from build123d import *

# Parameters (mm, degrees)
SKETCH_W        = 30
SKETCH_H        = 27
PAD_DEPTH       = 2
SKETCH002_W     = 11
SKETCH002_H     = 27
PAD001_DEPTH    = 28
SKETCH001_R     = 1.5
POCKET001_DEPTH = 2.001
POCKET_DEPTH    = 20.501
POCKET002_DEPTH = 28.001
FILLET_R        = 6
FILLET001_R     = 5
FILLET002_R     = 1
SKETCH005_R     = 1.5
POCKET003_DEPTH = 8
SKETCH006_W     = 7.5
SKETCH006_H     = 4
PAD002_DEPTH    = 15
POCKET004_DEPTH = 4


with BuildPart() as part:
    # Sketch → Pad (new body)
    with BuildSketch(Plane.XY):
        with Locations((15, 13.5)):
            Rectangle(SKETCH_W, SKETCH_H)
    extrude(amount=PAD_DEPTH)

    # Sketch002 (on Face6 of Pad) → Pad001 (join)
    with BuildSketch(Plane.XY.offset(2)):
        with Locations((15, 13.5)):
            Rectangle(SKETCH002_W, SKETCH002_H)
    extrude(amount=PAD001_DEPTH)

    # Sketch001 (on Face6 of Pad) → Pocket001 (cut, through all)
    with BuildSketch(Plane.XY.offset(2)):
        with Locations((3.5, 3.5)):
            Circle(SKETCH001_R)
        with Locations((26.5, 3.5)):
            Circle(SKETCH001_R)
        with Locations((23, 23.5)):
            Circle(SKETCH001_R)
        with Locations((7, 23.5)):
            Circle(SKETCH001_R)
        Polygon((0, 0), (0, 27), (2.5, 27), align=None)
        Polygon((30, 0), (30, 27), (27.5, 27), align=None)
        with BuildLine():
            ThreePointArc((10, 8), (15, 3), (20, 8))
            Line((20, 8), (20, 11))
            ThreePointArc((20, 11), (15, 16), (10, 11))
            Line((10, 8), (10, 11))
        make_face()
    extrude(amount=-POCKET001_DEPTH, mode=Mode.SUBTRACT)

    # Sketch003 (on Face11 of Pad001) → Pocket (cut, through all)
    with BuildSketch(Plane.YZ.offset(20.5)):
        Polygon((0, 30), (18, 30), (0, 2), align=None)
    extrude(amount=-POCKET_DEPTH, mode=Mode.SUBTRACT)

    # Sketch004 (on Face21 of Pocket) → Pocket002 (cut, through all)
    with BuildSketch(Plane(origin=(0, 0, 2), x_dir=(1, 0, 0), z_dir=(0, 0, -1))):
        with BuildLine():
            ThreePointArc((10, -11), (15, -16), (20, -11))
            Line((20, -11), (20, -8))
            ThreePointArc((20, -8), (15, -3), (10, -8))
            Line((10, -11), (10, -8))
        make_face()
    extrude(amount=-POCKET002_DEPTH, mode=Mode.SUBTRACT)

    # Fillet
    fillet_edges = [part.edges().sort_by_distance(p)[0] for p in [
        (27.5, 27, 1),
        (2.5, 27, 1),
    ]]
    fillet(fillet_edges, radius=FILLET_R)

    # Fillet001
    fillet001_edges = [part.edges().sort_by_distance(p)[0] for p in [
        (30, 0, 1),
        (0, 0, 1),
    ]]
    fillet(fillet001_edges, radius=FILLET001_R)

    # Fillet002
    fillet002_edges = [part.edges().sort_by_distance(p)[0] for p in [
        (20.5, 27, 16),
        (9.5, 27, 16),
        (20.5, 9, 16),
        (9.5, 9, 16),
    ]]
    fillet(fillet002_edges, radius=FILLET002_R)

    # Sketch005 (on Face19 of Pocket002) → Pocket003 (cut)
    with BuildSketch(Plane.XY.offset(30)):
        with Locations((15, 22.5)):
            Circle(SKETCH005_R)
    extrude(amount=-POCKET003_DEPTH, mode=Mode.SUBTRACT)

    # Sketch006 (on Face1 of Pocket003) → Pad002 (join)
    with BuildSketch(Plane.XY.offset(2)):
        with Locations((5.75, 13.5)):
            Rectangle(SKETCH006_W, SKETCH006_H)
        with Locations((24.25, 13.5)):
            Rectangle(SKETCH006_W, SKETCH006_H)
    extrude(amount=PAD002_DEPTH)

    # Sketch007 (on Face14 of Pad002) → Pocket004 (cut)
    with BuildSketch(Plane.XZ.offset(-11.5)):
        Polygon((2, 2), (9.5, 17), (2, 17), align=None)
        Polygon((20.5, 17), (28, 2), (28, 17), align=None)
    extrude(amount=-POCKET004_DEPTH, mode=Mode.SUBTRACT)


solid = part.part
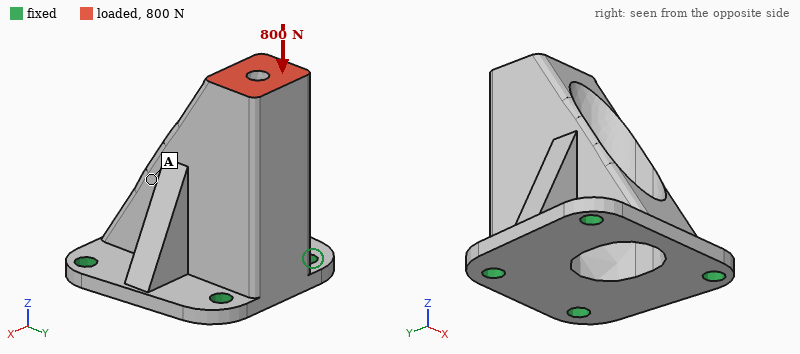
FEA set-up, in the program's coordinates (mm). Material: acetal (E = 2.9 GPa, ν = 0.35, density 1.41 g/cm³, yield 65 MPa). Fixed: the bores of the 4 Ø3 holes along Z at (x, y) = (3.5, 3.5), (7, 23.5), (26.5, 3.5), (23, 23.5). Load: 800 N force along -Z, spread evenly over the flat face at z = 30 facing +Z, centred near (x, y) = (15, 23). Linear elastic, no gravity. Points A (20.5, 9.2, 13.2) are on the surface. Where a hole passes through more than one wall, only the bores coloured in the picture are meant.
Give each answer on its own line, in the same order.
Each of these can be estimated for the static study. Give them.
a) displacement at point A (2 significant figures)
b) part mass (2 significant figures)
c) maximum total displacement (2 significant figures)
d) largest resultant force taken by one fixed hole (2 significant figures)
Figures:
0.073 mm
7.7 g
0.31 mm
410 N
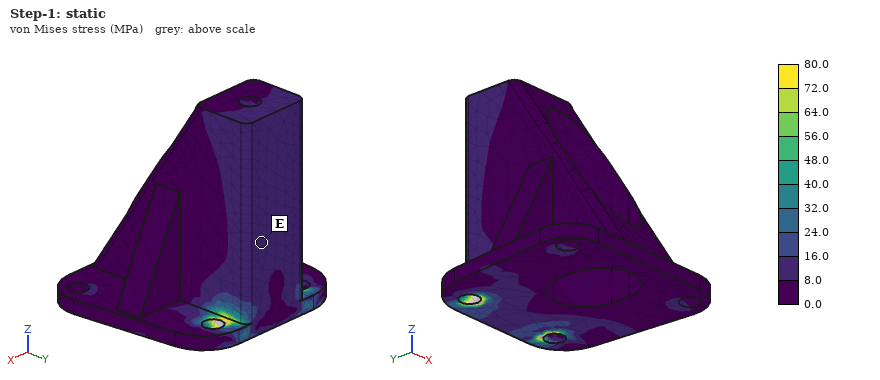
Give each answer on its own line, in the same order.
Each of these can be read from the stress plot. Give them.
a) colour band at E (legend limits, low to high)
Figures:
8.0 to 16.0 MPa
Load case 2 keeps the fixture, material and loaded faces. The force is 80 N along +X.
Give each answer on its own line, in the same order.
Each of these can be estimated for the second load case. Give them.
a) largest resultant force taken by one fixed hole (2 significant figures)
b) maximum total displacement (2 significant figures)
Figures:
130 N
0.28 mm
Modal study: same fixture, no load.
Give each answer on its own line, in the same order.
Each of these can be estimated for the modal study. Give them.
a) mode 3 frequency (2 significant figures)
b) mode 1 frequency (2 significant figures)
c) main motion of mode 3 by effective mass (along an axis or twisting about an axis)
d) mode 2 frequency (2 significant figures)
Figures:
5200 Hz
2200 Hz
along Z
2200 Hz
